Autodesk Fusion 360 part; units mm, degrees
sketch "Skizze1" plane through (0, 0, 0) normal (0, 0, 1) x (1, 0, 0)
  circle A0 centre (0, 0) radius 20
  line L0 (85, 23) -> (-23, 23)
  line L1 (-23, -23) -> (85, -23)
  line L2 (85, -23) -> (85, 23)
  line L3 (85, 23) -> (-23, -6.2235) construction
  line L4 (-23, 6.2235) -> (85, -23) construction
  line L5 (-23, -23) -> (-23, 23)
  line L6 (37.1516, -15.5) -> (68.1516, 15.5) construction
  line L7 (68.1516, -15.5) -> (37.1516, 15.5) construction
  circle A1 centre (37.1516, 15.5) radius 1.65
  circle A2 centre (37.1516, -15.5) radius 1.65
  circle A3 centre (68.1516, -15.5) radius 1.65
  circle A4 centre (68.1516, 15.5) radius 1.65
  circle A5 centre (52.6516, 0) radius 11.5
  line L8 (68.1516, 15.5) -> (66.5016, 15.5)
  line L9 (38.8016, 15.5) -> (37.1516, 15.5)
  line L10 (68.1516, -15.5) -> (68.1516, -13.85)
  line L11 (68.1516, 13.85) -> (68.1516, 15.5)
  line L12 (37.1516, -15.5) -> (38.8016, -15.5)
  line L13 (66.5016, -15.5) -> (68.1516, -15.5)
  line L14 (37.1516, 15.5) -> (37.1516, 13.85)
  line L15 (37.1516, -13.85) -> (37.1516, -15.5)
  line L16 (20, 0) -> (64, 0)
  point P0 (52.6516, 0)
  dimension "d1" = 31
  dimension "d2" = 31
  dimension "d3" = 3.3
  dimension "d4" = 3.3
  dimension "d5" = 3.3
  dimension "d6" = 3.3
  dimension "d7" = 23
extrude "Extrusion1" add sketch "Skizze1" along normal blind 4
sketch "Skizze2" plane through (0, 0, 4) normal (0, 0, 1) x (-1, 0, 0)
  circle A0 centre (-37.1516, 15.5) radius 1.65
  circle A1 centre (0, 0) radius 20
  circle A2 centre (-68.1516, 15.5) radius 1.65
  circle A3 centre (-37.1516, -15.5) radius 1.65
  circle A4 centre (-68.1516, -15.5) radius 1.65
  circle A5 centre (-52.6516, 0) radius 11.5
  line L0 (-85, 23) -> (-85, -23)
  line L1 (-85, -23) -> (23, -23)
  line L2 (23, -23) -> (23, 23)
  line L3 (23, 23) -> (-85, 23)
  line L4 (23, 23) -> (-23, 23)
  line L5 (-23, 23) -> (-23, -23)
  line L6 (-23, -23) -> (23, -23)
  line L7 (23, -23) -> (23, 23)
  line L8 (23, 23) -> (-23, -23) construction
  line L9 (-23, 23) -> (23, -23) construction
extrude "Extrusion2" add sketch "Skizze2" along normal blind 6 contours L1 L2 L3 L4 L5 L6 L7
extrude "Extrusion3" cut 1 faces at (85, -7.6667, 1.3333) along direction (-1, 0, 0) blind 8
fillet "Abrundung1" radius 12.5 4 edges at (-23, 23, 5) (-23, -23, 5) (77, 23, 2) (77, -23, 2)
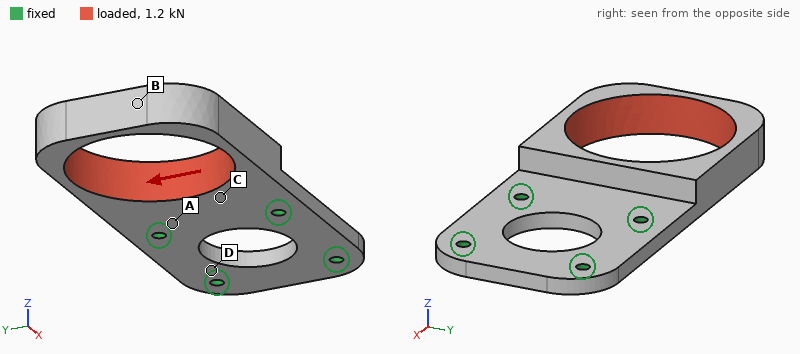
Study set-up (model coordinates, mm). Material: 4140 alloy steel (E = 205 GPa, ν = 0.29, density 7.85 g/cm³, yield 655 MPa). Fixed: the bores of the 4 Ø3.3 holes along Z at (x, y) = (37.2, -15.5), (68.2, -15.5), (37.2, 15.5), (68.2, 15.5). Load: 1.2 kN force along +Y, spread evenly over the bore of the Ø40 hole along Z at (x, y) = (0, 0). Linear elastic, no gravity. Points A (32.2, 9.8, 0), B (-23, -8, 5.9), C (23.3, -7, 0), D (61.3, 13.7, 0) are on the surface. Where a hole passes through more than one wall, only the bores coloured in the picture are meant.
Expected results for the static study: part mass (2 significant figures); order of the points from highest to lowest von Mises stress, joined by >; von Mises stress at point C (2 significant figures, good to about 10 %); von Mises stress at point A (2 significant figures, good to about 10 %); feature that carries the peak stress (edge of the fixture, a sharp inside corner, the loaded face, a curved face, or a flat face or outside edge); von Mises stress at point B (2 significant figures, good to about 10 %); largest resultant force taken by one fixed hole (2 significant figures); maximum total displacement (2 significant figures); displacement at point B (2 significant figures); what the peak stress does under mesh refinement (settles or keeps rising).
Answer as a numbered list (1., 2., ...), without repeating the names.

1. 120 g
2. B > C > A > D
3. 29 MPa
4. 16 MPa
5. edge of the fixture
6. 41 MPa
7. 1.3 kN
8. 61 µm
9. 60 µm
10. keeps rising
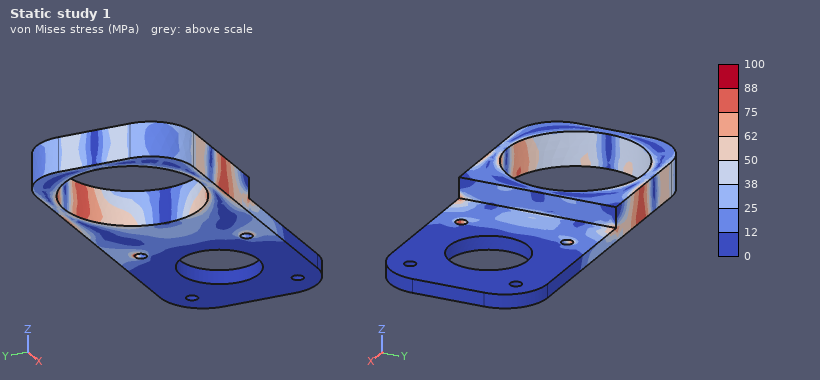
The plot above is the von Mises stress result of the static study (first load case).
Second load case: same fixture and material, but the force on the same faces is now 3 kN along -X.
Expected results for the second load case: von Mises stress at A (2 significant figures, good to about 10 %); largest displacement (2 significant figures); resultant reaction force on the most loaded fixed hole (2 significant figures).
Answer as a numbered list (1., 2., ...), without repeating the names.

1. 56 MPa
2. 0.18 mm
3. 1.4 kN
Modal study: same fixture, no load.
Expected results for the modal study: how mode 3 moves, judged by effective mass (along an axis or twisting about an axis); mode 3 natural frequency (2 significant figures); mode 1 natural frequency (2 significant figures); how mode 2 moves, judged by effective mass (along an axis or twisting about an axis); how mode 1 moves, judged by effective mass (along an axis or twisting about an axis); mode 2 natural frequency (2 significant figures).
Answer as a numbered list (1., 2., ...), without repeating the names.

1. along Y
2. 3200 Hz
3. 970 Hz
4. twisting about X
5. along Z
6. 2500 Hz
